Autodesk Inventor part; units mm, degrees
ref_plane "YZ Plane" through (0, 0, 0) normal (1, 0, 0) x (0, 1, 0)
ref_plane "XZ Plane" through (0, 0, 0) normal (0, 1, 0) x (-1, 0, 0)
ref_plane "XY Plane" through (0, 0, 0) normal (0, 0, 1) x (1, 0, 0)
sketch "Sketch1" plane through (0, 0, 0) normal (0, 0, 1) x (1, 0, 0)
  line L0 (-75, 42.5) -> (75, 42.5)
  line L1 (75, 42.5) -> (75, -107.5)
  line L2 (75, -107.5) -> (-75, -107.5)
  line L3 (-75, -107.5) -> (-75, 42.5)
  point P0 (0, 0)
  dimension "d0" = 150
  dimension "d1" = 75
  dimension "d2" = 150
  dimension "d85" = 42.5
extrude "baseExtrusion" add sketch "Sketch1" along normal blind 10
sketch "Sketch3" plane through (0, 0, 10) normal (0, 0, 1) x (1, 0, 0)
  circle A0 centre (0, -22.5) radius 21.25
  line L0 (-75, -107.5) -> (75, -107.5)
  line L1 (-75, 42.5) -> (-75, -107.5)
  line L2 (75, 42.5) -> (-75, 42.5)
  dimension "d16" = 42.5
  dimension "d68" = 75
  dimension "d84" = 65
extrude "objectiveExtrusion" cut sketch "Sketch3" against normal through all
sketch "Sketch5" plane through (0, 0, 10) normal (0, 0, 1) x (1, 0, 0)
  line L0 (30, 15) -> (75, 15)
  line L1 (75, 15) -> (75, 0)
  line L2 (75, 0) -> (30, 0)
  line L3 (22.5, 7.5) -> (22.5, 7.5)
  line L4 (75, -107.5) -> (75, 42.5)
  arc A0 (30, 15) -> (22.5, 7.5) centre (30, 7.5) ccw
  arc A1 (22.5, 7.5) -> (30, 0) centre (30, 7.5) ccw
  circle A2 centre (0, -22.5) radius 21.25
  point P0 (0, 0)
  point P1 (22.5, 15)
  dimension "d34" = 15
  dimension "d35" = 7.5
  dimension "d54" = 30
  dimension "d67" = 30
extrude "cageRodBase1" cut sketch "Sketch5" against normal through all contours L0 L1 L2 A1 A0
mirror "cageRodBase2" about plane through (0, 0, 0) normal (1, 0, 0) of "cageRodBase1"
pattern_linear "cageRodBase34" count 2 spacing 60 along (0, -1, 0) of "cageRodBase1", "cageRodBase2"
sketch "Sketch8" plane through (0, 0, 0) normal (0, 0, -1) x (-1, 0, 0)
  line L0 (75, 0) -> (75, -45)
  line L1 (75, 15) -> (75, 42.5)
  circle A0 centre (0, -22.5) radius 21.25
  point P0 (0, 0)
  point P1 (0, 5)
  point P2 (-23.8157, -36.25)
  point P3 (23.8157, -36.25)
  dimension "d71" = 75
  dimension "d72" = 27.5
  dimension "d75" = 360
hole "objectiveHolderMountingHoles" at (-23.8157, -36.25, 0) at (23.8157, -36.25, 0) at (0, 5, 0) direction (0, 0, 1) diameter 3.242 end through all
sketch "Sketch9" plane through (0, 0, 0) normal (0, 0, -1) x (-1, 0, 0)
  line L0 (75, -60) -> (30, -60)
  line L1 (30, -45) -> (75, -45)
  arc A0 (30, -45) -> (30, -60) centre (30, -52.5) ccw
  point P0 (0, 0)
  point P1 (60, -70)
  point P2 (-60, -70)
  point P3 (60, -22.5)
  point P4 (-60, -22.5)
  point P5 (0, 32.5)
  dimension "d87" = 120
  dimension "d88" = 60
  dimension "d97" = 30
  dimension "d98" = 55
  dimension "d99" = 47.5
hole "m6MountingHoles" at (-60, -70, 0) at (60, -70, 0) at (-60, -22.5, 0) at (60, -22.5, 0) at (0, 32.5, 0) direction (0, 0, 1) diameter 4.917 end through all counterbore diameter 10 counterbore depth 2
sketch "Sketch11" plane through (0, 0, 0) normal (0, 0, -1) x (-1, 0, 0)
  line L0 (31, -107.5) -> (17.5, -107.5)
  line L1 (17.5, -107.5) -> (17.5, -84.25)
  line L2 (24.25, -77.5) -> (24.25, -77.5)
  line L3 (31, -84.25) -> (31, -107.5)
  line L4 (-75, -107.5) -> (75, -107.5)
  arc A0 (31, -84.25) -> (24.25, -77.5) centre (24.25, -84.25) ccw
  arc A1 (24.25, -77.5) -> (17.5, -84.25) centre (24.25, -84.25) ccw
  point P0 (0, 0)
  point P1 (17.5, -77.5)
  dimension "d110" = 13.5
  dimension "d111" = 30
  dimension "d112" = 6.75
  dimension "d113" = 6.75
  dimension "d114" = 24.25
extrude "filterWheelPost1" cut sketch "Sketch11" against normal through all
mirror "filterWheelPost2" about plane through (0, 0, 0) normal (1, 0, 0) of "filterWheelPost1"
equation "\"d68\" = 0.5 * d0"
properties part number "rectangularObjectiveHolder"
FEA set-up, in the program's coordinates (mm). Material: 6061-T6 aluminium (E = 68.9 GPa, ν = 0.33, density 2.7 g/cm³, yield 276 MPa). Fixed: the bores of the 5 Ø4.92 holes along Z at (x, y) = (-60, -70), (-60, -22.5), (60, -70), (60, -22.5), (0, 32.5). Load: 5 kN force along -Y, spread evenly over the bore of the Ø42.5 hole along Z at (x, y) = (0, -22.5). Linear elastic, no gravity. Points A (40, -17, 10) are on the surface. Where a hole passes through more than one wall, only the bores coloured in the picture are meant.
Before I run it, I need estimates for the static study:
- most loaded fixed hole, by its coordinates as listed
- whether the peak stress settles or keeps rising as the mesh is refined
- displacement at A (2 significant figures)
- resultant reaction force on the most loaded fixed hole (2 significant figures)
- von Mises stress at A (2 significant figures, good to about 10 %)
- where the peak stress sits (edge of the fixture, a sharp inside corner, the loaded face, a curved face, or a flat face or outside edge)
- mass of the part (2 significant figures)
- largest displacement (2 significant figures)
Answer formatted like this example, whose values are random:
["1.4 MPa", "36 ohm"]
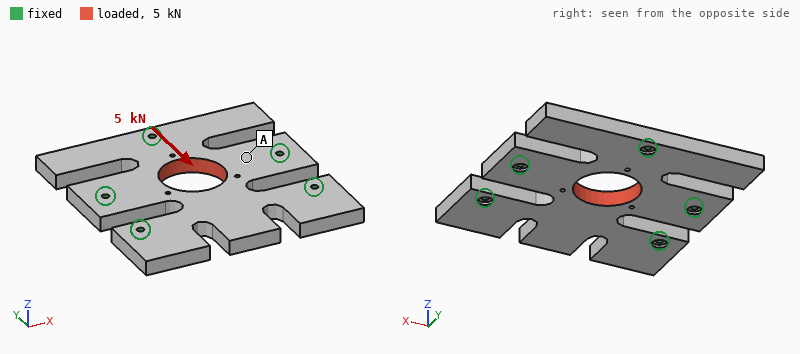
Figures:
["(0, 32.5)", "keeps rising", "6.2 µm", "2.9 kN", "3.8 MPa", "edge of the fixture", "460 g", "14 µm"]
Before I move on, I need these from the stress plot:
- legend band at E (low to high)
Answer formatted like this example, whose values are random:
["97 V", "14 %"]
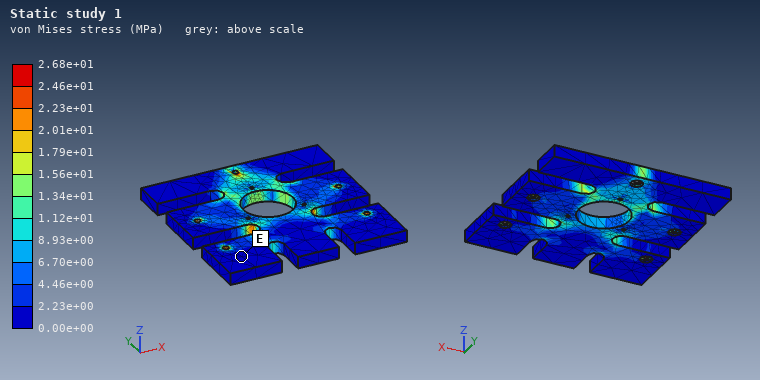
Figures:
["0.00e+00 to 2.23e+00 MPa"]
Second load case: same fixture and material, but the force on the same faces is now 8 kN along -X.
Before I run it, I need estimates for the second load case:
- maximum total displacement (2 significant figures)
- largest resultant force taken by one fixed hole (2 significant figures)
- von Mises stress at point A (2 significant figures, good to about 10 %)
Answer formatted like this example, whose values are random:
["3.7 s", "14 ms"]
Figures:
["20 µm", "3.0 kN", "9.7 MPa"]
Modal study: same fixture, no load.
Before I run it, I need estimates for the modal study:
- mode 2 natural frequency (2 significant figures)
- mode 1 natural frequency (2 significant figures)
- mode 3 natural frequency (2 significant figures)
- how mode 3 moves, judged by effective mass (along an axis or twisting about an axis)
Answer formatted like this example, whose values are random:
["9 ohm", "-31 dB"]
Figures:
["1600 Hz", "1400 Hz", "2100 Hz", "along Z"]
